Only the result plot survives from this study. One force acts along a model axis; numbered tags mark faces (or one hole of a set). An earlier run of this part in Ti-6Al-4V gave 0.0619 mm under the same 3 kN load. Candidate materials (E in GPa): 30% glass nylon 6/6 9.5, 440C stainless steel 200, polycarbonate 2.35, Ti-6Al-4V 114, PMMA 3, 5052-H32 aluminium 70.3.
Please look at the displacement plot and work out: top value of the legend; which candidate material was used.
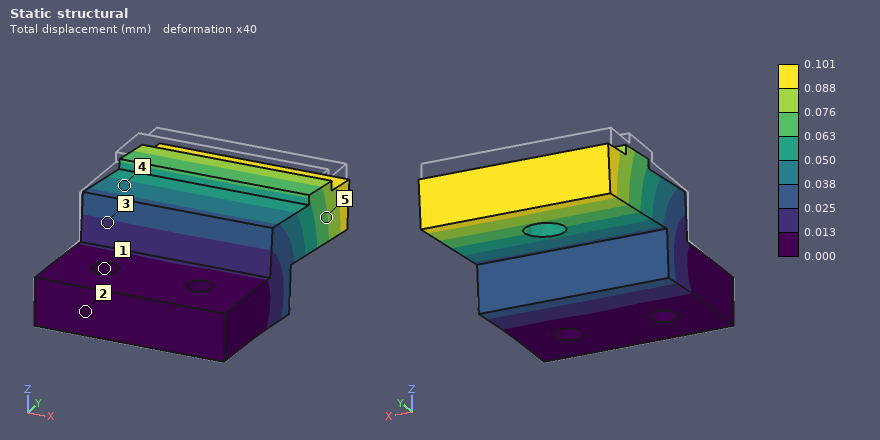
0.101 mm
5052-H32 aluminium
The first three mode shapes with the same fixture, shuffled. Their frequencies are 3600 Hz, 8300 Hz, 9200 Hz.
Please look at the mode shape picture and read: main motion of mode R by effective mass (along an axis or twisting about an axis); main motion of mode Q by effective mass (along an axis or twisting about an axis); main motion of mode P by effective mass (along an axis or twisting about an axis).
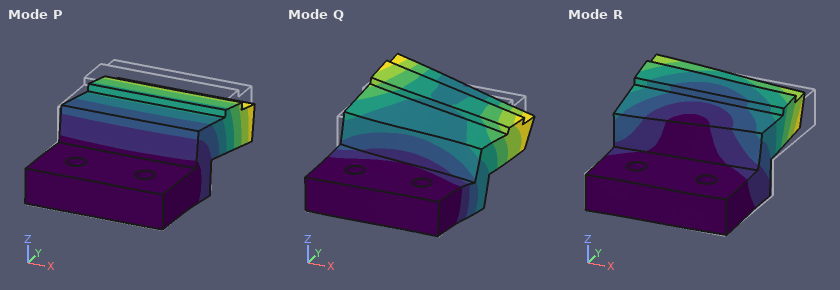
along X
along X
along Z
